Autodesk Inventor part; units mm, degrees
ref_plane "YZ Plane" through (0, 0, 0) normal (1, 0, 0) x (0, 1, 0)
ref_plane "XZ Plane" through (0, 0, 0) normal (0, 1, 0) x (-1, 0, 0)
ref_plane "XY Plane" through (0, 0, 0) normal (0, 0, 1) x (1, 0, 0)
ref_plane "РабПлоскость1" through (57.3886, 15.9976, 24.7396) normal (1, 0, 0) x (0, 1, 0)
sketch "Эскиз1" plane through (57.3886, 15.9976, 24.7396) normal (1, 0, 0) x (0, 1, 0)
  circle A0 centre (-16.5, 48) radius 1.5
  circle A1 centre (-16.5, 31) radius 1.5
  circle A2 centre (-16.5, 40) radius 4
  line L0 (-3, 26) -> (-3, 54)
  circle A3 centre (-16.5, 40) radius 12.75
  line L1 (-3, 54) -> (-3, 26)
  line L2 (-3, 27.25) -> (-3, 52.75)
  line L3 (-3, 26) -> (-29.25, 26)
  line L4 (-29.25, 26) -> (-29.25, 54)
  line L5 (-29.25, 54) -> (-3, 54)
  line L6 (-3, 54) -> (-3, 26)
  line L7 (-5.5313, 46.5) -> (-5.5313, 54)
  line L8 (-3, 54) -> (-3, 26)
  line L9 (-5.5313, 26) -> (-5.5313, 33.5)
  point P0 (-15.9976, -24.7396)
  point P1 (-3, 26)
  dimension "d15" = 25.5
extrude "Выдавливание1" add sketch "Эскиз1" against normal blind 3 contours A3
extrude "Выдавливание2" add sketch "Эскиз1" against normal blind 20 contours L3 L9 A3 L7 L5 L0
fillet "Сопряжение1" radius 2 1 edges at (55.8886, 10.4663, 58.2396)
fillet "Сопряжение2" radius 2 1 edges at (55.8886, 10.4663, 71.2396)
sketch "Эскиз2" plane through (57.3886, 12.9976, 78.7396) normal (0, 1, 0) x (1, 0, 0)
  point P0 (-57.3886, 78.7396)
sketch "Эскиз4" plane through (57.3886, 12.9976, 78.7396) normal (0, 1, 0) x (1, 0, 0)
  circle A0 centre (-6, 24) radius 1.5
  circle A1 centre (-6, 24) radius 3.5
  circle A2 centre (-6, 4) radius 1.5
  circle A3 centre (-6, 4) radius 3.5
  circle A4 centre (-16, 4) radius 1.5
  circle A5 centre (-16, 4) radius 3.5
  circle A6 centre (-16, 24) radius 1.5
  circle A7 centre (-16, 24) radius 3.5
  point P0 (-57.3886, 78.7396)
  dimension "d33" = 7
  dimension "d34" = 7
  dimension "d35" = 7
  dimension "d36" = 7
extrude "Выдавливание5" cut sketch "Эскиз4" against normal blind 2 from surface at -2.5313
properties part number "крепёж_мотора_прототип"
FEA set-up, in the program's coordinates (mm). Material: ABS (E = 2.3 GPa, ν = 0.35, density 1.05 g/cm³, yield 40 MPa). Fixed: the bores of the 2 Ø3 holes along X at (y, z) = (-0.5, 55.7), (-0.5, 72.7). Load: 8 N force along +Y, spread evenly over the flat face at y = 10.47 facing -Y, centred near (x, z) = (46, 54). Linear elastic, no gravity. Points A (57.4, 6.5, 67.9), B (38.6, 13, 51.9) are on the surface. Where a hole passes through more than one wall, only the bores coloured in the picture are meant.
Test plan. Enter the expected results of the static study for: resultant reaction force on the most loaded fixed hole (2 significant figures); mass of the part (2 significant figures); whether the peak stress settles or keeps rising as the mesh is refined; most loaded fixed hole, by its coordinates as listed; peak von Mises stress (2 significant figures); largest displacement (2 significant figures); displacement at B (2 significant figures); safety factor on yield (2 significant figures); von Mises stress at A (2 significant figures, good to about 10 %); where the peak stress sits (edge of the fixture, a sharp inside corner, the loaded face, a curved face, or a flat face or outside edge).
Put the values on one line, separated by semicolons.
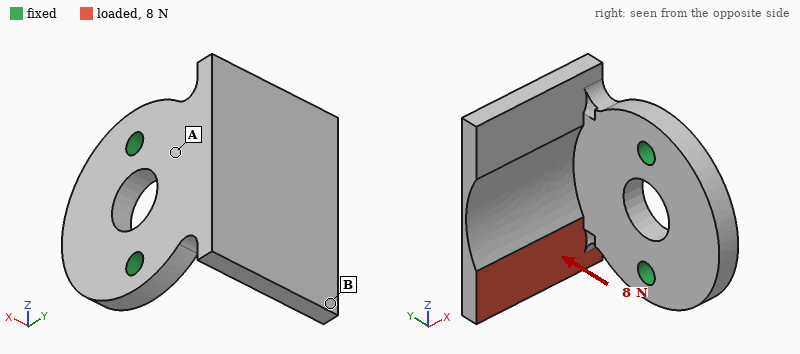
8.7 N; 2.6 g; settles; (-0.5, 55.7); 12 MPa; 0.44 mm; 0.40 mm; 3.4; 2.0 MPa; a curved face
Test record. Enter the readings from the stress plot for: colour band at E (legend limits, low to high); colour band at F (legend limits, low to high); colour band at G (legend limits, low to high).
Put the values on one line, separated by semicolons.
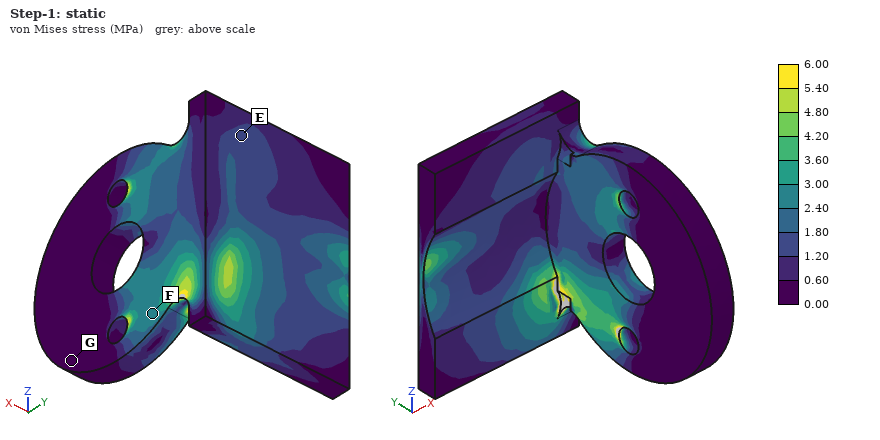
1.20 to 1.80 MPa; 2.40 to 3.00 MPa; 0.00 to 0.60 MPa
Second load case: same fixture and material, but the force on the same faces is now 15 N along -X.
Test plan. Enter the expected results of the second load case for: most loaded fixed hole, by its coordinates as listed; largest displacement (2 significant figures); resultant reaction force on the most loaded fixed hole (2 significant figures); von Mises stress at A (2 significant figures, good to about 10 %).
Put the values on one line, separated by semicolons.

(-0.5, 55.7); 0.25 mm; 16 N; 2.8 MPa
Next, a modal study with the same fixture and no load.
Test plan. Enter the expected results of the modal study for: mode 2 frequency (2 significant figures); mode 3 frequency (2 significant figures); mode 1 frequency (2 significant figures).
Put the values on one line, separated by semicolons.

1500 Hz; 2200 Hz; 940 Hz
